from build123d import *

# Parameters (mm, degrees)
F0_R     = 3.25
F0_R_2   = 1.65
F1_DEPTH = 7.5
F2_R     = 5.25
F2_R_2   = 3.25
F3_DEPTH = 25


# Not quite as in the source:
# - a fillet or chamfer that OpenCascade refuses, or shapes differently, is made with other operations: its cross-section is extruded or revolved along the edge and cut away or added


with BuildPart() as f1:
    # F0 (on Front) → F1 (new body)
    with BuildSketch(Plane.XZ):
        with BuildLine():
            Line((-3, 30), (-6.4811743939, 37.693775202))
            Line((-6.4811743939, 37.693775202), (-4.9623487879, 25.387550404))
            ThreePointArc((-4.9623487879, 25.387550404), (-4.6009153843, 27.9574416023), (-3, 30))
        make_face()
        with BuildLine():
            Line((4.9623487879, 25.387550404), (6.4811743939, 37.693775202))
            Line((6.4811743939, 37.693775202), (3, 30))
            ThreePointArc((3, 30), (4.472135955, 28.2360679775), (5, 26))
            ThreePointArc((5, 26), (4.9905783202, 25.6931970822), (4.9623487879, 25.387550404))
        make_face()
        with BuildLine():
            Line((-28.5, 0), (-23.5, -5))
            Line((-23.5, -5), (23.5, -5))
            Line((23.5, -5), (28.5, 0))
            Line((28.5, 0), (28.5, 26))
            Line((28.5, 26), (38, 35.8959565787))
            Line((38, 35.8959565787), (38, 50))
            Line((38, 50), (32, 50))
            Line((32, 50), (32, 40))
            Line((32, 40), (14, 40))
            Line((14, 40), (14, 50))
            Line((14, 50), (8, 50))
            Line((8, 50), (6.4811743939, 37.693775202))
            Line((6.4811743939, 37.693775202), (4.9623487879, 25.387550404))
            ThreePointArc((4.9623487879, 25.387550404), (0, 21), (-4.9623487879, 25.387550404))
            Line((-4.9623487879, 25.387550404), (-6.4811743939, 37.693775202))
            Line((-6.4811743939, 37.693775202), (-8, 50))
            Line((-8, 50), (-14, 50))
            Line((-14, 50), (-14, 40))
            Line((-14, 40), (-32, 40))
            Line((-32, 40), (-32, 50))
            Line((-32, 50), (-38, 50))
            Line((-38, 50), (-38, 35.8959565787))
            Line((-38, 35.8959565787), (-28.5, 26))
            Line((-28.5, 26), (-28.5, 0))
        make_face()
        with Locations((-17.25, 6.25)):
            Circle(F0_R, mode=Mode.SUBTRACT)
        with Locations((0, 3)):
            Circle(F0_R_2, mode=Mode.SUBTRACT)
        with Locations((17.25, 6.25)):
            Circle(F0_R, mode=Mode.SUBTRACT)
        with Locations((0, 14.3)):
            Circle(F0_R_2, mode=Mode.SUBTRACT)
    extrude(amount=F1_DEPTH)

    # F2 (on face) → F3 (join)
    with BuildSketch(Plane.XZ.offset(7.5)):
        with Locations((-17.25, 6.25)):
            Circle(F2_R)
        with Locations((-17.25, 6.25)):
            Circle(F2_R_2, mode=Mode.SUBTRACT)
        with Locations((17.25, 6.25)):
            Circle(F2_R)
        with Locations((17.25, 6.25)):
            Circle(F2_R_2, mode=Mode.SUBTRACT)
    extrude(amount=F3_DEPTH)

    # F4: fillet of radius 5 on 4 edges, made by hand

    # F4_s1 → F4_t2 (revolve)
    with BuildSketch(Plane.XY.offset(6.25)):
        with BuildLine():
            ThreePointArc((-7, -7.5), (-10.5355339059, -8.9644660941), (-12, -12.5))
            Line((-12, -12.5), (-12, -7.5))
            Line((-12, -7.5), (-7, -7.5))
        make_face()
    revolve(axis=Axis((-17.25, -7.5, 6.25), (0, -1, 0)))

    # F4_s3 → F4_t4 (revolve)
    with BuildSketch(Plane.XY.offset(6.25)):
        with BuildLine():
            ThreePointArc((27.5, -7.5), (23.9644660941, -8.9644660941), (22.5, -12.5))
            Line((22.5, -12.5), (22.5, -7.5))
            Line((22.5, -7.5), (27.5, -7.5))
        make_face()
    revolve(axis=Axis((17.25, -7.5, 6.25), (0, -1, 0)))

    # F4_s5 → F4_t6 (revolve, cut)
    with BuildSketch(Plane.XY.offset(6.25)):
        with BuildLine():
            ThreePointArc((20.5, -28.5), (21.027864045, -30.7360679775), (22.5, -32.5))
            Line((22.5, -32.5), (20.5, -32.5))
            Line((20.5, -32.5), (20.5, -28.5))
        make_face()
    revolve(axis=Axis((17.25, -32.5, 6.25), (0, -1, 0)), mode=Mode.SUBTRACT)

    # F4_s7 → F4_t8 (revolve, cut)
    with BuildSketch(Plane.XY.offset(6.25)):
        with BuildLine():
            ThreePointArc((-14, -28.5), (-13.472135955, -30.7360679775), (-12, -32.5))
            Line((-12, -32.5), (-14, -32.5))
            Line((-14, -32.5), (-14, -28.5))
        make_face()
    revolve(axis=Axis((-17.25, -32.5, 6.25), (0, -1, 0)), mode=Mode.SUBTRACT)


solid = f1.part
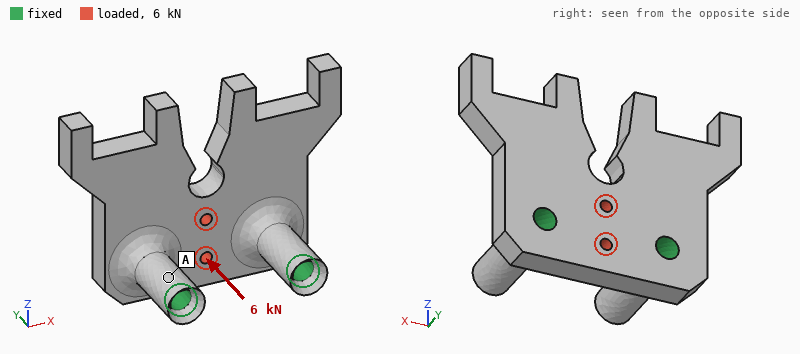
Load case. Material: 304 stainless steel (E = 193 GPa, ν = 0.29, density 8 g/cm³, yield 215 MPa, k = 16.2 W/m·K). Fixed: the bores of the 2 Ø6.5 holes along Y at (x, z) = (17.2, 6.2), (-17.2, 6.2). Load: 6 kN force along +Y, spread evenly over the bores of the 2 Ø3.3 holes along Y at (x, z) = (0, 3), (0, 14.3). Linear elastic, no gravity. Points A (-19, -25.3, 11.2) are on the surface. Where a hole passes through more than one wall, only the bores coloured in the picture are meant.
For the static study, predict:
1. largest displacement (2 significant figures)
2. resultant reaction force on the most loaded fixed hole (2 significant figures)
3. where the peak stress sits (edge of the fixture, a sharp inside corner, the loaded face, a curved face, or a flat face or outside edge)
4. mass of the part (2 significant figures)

11 µm
3.1 kN
the loaded face
190 g
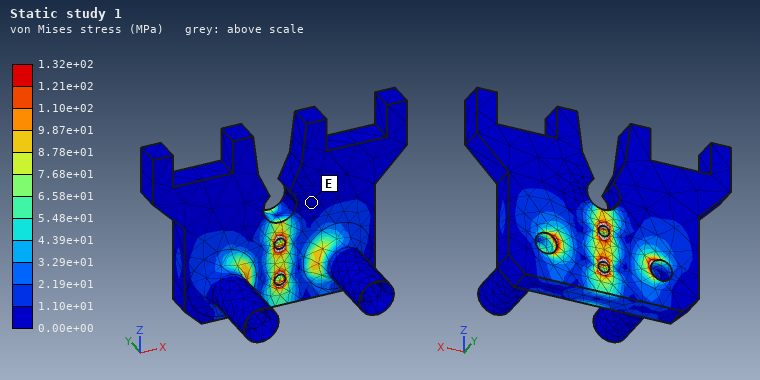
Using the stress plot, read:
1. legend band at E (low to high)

0.00e+00 to 1.10e+01 MPa
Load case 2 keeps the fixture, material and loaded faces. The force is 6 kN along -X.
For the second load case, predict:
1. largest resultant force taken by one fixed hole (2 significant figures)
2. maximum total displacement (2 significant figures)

3.0 kN
2.6 µm
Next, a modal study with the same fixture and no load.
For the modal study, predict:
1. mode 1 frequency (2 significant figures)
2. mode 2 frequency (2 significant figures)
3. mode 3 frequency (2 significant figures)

4100 Hz
4200 Hz
7900 Hz
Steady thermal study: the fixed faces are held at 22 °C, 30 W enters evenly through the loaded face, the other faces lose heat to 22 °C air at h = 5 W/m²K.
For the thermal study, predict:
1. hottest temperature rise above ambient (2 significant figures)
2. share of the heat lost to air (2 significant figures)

82 K
3.2 %
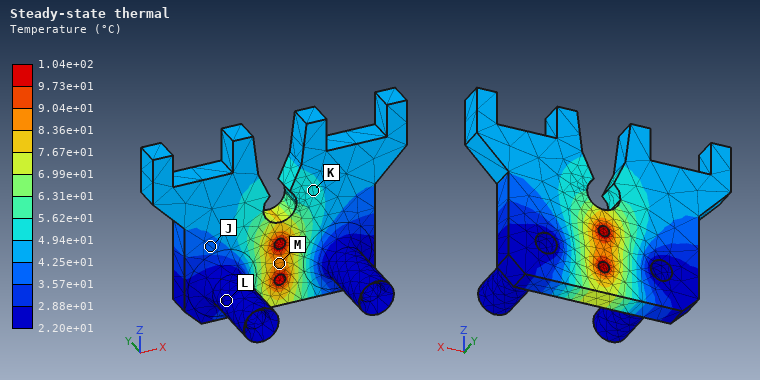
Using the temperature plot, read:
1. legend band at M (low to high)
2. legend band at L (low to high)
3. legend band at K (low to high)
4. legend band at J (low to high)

8.36e+01 to 9.04e+01 °C
2.20e+01 to 2.88e+01 °C
4.94e+01 to 5.62e+01 °C
3.57e+01 to 4.25e+01 °C
